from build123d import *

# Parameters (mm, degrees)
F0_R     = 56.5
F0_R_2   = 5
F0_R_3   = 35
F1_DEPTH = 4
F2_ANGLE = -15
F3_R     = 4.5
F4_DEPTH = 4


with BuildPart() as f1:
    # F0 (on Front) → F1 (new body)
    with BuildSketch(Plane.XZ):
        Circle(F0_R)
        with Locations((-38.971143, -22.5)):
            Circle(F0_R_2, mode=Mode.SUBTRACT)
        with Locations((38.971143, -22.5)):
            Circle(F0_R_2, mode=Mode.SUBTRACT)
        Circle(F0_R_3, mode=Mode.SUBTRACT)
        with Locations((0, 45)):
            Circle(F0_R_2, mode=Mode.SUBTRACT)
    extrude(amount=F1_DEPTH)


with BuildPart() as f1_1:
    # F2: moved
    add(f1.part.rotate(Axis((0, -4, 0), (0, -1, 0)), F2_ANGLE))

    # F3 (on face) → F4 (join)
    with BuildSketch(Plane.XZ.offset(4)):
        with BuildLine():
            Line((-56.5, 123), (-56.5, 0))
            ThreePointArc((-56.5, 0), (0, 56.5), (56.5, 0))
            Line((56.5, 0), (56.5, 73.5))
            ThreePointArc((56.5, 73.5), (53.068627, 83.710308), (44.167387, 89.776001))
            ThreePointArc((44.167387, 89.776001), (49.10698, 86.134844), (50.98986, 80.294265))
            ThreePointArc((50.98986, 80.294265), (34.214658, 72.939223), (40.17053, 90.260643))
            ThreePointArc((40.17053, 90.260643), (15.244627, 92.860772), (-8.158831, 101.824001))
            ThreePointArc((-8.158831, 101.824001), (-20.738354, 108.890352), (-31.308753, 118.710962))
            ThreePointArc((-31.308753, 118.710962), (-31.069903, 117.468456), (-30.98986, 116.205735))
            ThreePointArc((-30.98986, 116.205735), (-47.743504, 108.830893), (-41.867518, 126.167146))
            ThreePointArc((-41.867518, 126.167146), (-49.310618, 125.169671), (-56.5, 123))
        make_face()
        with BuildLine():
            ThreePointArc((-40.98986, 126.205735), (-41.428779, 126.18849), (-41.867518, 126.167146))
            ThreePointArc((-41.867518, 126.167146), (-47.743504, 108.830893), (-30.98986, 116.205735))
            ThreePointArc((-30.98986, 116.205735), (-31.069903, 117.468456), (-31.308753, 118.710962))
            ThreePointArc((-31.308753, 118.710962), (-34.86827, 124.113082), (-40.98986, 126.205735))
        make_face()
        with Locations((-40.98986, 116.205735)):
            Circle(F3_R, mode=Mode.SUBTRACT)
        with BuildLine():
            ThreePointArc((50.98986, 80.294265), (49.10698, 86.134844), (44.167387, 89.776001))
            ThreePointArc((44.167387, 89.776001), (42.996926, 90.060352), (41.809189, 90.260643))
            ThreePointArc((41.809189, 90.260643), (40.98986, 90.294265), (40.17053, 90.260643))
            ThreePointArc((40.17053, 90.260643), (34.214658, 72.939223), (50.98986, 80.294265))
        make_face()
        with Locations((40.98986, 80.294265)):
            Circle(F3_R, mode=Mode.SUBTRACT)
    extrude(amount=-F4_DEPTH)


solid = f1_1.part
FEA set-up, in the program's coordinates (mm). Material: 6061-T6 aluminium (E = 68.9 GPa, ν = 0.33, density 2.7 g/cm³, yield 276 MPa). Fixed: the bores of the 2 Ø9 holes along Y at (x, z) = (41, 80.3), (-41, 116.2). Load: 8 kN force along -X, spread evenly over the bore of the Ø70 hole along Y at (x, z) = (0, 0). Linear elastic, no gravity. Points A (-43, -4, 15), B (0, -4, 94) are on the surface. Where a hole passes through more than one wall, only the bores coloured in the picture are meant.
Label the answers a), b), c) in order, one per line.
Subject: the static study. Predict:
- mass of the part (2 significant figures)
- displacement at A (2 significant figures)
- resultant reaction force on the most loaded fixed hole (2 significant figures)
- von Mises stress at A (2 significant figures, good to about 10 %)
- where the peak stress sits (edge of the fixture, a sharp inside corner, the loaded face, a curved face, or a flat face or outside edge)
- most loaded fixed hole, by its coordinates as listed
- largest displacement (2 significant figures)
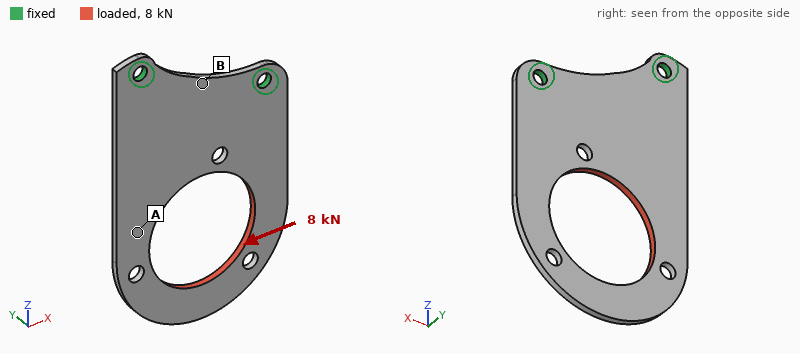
a) 130 g
b) 0.21 mm
c) 10 kN
d) 54 MPa
e) edge of the fixture
f) (41, 80.3)
g) 0.52 mm
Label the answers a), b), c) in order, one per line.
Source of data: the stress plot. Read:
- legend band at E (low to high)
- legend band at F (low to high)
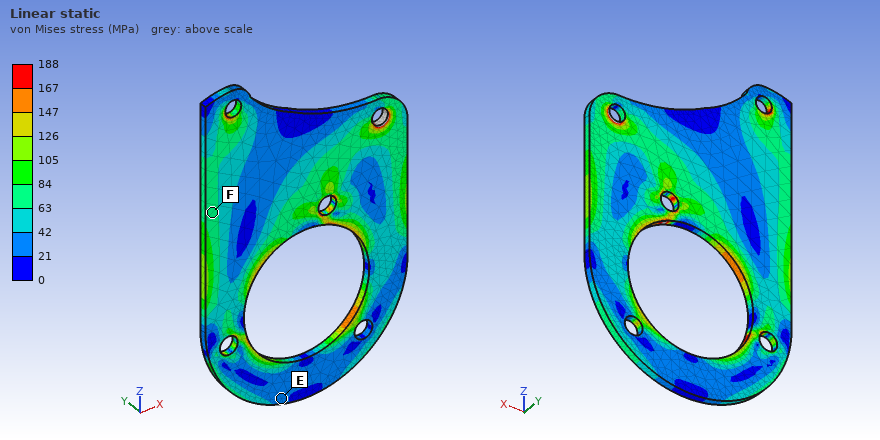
a) 21 to 42 MPa
b) 63 to 84 MPa
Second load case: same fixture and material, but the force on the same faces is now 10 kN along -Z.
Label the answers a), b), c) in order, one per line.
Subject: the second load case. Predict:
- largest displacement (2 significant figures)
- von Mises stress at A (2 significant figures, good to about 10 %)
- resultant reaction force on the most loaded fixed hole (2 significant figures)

a) 0.13 mm
b) 42 MPa
c) 5.2 kN
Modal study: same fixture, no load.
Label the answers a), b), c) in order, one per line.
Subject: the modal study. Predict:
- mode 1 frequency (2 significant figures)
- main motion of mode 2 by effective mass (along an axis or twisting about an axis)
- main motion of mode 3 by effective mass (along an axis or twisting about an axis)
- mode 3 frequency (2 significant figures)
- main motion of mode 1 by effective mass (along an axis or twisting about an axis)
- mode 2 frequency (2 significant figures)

a) 190 Hz
b) twisting about Z
c) along Y
d) 820 Hz
e) along Y
f) 470 Hz
